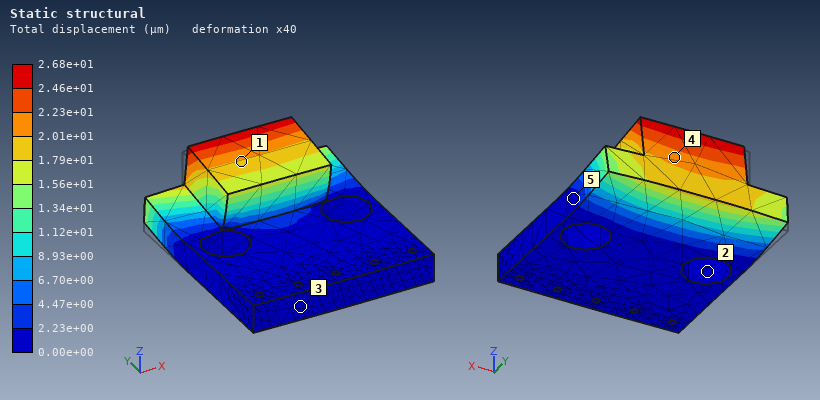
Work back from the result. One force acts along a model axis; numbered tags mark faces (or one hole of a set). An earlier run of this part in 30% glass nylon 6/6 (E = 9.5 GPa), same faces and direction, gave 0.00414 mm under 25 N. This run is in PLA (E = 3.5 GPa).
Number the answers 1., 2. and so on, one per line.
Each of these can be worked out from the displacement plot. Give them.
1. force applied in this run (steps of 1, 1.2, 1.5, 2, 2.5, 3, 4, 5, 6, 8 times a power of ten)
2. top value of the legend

1. 60 N
2. 2.68e+01 µm
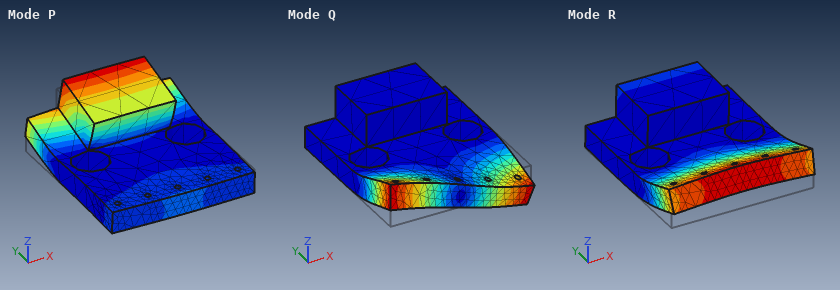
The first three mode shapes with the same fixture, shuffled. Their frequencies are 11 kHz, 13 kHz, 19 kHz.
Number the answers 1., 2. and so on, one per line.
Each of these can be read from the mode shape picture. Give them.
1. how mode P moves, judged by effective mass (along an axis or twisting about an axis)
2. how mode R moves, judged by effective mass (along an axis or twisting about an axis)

1. along Z
2. along Z
